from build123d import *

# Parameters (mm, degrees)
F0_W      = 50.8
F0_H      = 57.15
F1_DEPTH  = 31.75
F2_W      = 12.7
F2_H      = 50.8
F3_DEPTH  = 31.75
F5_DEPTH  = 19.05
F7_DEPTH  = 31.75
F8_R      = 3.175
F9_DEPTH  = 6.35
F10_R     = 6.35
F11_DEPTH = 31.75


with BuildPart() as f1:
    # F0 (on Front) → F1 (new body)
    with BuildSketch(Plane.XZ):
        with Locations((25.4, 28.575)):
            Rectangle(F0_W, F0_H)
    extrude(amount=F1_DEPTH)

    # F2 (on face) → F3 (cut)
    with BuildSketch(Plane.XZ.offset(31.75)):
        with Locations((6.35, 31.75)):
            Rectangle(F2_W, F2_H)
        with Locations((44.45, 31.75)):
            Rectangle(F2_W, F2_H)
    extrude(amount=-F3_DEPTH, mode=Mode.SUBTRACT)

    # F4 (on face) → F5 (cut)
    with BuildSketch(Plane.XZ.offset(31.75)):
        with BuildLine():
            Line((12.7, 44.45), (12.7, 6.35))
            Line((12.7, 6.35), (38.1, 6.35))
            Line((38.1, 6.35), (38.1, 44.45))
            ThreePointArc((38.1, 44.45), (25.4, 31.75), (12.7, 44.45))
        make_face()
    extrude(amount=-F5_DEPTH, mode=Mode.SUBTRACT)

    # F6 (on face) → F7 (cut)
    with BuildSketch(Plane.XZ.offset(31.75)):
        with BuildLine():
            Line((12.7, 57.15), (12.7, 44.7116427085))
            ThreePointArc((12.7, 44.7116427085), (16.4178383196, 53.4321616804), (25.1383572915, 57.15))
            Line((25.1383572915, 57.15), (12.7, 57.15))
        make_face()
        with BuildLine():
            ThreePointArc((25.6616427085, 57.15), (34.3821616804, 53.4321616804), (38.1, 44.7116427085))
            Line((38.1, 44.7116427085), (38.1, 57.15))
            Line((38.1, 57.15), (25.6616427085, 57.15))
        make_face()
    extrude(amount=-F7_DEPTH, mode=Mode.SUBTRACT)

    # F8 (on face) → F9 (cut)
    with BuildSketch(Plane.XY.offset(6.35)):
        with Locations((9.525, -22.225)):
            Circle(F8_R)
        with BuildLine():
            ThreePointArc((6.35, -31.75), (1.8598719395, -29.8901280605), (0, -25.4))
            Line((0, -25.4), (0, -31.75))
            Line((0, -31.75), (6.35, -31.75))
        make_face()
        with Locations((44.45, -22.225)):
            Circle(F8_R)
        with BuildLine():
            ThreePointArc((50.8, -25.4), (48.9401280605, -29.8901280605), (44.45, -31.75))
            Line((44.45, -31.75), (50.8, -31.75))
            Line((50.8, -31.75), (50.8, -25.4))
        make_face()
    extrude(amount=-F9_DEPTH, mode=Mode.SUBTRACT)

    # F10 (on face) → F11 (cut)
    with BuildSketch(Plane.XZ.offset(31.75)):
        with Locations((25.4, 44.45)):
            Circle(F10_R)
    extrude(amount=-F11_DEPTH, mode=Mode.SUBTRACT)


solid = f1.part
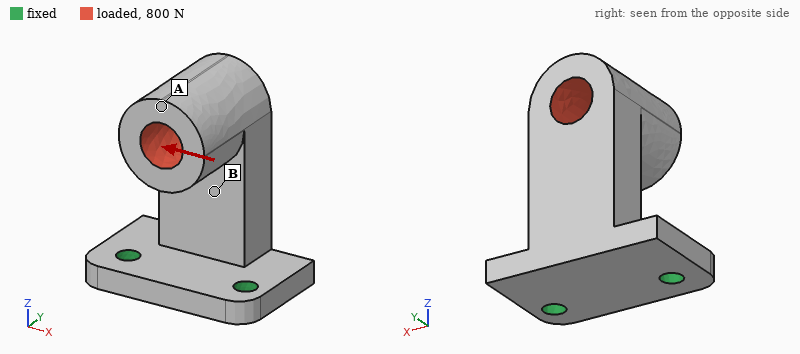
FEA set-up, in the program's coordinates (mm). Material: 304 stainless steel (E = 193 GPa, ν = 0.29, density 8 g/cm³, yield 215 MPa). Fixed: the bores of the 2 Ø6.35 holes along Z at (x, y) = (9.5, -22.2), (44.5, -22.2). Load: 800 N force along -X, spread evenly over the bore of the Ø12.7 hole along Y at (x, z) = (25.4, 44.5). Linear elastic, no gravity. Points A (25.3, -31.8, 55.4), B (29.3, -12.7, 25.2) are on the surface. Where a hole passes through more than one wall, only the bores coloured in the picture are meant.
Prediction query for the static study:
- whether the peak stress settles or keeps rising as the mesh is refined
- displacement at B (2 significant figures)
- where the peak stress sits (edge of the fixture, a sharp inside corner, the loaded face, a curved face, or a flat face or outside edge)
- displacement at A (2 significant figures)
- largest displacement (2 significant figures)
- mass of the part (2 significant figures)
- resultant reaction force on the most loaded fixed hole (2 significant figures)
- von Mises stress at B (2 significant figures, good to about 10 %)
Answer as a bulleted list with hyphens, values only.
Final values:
- keeps rising
- 14 µm
- edge of the fixture
- 42 µm
- 43 µm
- 250 g
- 1.1 kN
- 20 MPa
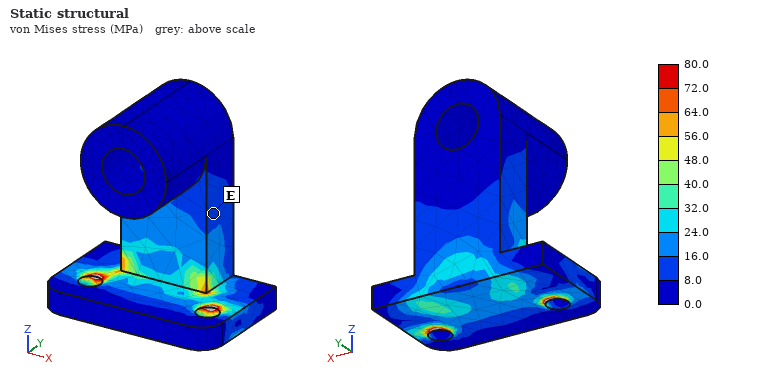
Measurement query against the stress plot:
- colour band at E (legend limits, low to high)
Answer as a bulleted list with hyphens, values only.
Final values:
- 8.0 to 16.0 MPa
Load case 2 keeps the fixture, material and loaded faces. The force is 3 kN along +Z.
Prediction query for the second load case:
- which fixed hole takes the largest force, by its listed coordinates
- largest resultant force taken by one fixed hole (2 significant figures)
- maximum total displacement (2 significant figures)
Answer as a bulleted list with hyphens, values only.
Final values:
- (9.5, -22.2)
- 1.6 kN
- 60 µm
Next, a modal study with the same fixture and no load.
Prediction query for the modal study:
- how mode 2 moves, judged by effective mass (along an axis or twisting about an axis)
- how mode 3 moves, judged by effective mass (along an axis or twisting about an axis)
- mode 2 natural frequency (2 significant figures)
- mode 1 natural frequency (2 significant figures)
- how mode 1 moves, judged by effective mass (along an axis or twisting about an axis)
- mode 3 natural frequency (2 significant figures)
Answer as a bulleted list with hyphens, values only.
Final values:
- along X
- along Z
- 2400 Hz
- 1200 Hz
- along Y
- 5100 Hz
